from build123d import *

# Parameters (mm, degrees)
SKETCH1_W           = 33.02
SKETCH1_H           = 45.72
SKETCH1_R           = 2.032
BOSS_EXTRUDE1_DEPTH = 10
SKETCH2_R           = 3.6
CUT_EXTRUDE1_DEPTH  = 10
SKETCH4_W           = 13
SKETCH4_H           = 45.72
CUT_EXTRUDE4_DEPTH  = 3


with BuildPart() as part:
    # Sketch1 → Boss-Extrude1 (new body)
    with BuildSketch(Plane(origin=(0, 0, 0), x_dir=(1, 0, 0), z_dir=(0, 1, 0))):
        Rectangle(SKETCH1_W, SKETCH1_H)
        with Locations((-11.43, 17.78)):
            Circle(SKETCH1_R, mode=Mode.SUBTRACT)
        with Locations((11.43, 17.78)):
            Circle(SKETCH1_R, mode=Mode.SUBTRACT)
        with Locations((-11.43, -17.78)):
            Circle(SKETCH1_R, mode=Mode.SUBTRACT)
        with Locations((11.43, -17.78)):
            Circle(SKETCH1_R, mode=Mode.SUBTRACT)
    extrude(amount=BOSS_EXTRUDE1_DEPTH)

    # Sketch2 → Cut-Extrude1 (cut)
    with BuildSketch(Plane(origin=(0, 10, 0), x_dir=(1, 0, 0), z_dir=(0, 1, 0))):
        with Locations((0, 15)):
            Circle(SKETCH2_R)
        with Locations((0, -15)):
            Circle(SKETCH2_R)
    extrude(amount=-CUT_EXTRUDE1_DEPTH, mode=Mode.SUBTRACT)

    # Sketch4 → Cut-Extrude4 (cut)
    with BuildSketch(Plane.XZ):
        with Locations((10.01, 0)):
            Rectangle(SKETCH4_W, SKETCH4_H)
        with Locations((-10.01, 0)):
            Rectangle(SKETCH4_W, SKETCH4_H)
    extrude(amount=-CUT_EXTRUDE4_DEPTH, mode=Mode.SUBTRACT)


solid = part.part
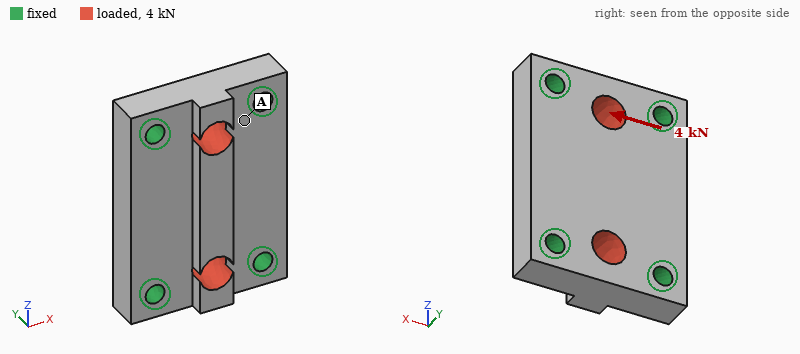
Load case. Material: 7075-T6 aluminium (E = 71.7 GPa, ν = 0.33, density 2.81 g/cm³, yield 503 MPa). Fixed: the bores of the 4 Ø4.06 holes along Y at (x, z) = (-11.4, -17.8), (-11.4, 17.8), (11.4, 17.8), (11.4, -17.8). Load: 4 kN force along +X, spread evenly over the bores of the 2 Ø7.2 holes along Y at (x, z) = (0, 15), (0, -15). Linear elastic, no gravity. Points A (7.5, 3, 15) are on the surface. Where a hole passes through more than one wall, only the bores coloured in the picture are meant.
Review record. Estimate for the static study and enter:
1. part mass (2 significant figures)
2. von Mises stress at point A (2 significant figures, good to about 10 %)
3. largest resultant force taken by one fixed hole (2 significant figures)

29 g
19 MPa
1.0 kN
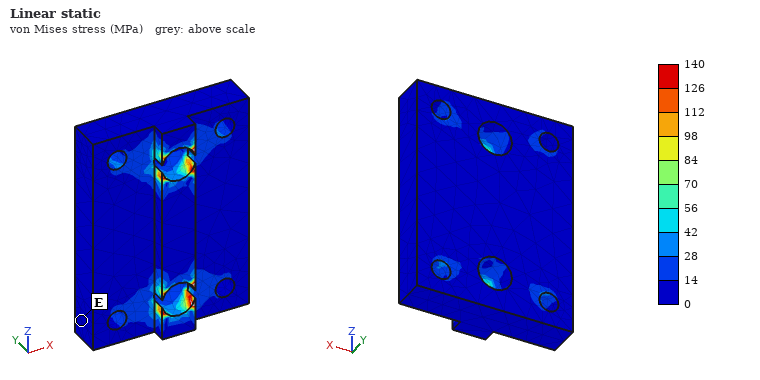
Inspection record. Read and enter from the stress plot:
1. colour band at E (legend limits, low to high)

0 to 14 MPa
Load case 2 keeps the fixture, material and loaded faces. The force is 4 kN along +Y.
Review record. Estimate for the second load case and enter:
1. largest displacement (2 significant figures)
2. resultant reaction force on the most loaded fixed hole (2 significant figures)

13 µm
1.0 kN
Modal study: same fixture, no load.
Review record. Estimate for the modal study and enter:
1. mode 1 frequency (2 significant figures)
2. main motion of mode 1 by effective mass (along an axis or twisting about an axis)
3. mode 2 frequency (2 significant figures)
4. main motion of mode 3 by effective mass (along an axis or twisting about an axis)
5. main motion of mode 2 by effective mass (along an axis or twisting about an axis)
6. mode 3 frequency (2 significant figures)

22 kHz
along Y
29 kHz
along X
twisting about Z
34 kHz
